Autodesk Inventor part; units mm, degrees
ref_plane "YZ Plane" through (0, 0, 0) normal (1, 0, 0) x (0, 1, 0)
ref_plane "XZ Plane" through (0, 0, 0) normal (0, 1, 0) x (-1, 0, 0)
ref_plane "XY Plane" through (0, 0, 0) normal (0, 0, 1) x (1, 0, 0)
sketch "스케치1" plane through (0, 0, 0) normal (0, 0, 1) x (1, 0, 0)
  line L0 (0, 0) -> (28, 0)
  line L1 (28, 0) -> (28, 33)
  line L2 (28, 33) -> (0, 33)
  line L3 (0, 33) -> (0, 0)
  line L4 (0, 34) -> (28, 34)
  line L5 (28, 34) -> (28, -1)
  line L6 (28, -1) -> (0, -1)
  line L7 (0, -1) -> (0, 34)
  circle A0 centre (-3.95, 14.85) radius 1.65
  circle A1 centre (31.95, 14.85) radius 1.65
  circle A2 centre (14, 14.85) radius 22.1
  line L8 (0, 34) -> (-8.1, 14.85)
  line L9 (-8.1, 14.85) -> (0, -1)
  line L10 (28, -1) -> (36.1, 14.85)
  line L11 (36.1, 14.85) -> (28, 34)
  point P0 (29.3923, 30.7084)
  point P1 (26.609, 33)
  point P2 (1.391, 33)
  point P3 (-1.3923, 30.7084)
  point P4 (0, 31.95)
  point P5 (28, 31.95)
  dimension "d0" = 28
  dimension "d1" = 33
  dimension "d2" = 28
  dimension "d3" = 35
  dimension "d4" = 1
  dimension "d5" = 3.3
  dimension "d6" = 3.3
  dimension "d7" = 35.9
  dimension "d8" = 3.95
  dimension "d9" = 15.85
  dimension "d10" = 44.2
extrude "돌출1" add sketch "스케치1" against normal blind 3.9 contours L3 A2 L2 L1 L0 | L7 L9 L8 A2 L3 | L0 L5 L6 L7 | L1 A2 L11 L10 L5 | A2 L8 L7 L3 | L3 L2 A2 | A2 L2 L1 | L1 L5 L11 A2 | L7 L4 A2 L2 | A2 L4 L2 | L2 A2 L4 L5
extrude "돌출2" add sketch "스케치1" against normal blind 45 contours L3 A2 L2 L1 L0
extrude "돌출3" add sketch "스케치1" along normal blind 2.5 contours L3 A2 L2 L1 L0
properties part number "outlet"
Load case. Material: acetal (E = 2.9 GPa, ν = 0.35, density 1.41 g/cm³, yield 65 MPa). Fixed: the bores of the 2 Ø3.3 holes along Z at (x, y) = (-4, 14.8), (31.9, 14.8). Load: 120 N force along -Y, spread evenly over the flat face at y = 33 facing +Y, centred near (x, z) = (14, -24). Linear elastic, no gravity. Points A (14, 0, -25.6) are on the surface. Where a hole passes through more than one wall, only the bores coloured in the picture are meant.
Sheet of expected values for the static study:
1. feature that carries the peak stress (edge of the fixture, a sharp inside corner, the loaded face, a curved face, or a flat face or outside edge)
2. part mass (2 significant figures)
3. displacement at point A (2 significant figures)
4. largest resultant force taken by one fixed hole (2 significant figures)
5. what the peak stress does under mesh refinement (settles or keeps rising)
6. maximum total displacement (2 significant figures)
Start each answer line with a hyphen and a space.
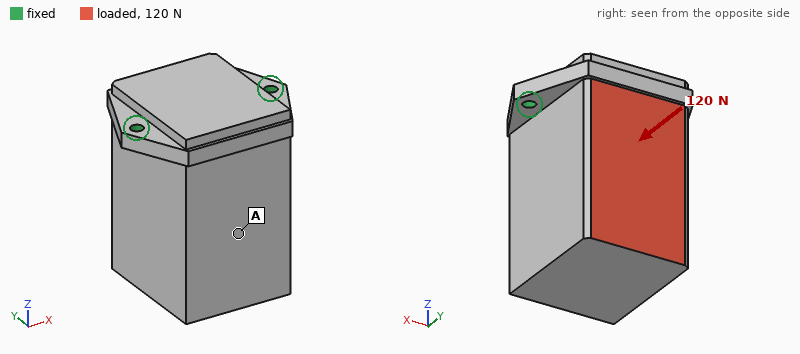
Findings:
- edge of the fixture
- 64 g
- 0.49 mm
- 60 N
- keeps rising
- 0.82 mm
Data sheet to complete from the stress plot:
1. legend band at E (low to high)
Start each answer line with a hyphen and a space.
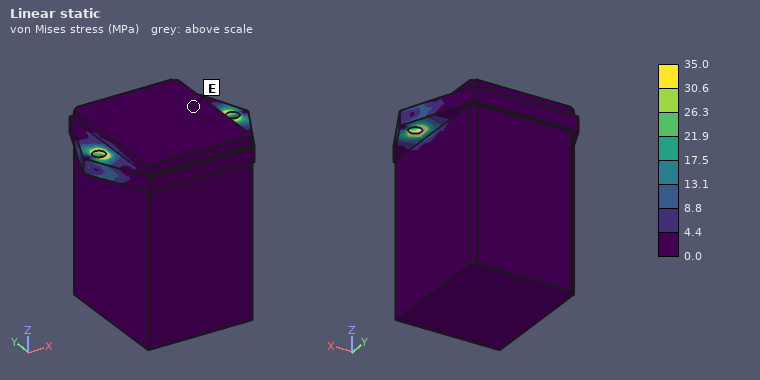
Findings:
- 0.0 to 4.4 MPa
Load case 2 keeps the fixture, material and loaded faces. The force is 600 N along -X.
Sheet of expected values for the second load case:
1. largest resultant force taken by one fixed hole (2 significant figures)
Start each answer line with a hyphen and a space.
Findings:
- 600 N
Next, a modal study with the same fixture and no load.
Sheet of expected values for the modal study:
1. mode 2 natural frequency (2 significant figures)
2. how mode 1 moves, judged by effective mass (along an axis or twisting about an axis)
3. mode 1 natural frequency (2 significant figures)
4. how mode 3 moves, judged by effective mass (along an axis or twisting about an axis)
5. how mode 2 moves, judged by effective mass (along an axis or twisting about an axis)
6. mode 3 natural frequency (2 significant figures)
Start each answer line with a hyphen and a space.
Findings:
- 1200 Hz
- along Y
- 310 Hz
- along Z
- along X
- 2000 Hz
